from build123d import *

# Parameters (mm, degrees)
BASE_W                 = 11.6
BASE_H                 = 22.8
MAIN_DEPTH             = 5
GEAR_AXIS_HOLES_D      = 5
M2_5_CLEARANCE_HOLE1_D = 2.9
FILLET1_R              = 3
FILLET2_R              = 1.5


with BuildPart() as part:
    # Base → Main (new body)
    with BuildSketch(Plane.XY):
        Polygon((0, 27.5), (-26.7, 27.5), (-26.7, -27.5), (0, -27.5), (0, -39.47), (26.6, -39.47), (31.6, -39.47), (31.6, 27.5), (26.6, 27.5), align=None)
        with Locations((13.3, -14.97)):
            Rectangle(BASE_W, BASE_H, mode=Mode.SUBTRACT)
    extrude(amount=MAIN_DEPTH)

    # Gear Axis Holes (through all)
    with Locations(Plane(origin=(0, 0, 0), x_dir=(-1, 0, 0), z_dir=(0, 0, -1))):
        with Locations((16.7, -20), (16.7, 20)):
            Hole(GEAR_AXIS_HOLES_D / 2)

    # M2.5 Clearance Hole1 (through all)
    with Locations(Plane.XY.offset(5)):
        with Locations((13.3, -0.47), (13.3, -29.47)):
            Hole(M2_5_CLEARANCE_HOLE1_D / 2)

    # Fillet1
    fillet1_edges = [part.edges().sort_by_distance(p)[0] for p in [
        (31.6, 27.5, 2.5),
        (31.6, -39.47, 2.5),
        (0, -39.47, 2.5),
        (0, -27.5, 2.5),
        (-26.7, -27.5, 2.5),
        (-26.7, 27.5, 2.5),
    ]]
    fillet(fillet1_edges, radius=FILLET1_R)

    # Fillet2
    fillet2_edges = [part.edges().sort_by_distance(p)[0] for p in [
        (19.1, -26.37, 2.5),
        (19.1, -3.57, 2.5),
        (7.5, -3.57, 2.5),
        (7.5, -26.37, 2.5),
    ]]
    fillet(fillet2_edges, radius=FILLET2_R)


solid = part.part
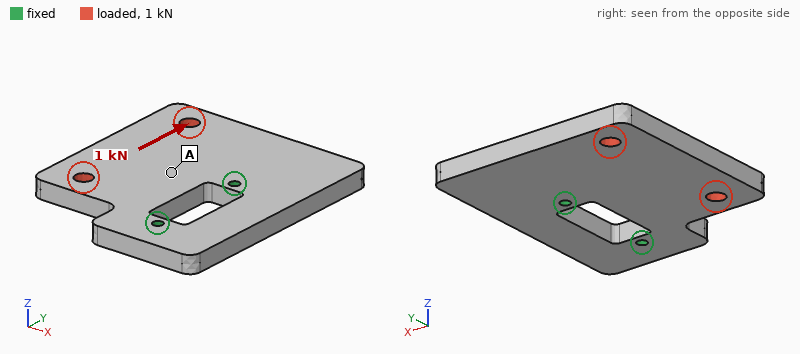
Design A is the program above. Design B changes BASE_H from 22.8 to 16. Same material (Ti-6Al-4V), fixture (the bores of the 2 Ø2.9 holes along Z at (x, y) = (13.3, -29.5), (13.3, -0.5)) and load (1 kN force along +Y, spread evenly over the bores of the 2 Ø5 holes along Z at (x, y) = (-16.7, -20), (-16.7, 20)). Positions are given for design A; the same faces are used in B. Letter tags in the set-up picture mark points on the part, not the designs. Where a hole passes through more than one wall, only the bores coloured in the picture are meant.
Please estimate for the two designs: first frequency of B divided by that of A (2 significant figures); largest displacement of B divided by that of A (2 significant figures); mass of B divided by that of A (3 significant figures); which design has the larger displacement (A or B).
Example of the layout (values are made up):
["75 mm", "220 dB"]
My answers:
["1.1", "0.82", "1.02", "A"]
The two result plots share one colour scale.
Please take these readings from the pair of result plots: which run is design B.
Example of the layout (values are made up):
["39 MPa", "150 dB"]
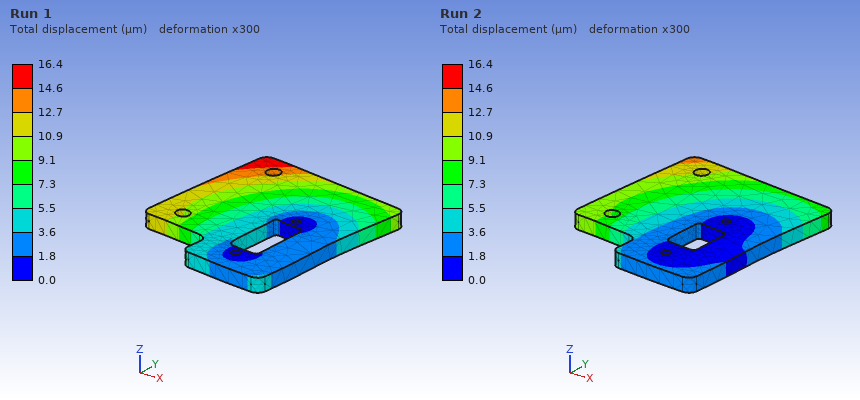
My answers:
["Run 2"]
